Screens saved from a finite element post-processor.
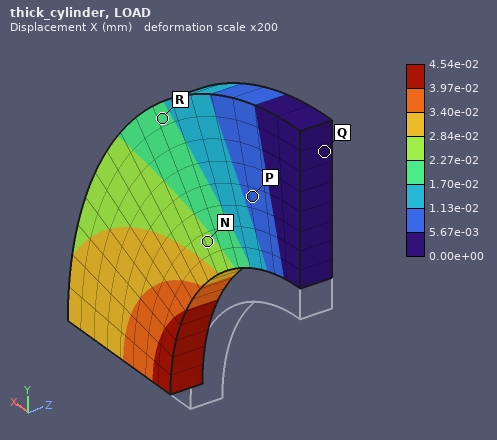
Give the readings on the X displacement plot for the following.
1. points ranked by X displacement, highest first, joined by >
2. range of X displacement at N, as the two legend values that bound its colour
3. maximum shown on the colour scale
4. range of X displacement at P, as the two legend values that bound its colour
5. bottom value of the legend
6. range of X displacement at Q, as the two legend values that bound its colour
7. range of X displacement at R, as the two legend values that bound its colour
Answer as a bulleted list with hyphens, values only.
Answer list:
- N > R > P > Q
- 2.27e-02 to 2.84e-02 mm
- 4.54e-02 mm
- 5.67e-03 to 1.13e-02 mm
- 0.00e+00 mm
- 0.00e+00 to 5.67e-03 mm
- 1.70e-02 to 2.27e-02 mm
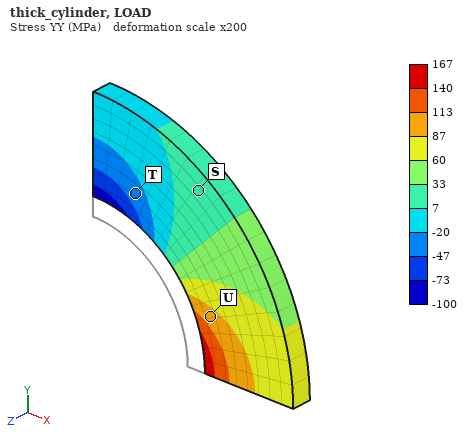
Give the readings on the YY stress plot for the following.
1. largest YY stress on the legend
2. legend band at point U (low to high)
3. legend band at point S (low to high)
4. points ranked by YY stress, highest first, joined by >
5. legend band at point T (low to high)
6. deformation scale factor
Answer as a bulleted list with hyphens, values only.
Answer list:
- 167 MPa
- 87 to 113 MPa
- 7 to 33 MPa
- U > S > T
- -47 to -20 MPa
- 200
